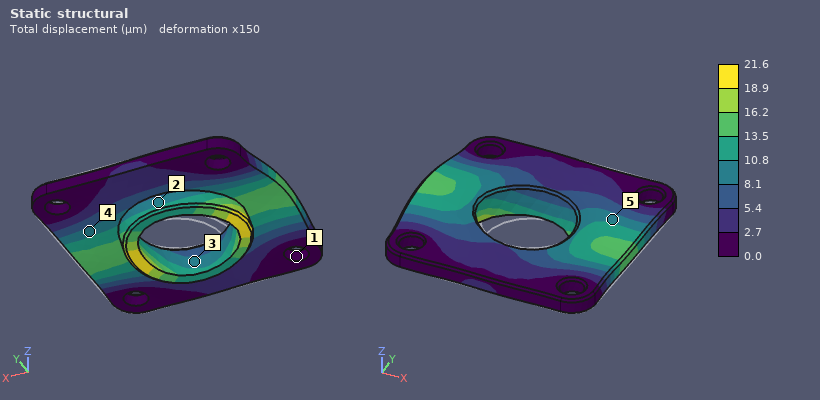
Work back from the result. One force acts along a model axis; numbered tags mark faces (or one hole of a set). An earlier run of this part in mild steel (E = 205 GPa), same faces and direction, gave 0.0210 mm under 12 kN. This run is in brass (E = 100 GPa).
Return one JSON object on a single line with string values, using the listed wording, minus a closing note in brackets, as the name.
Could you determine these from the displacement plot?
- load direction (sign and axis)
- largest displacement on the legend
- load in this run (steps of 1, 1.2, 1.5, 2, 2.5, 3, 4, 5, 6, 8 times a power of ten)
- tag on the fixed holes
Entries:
{"load direction": "-X", "largest displacement on the legend": "21.6 µm", "load in this run": "6 kN", "tag on the fixed holes": "1"}
